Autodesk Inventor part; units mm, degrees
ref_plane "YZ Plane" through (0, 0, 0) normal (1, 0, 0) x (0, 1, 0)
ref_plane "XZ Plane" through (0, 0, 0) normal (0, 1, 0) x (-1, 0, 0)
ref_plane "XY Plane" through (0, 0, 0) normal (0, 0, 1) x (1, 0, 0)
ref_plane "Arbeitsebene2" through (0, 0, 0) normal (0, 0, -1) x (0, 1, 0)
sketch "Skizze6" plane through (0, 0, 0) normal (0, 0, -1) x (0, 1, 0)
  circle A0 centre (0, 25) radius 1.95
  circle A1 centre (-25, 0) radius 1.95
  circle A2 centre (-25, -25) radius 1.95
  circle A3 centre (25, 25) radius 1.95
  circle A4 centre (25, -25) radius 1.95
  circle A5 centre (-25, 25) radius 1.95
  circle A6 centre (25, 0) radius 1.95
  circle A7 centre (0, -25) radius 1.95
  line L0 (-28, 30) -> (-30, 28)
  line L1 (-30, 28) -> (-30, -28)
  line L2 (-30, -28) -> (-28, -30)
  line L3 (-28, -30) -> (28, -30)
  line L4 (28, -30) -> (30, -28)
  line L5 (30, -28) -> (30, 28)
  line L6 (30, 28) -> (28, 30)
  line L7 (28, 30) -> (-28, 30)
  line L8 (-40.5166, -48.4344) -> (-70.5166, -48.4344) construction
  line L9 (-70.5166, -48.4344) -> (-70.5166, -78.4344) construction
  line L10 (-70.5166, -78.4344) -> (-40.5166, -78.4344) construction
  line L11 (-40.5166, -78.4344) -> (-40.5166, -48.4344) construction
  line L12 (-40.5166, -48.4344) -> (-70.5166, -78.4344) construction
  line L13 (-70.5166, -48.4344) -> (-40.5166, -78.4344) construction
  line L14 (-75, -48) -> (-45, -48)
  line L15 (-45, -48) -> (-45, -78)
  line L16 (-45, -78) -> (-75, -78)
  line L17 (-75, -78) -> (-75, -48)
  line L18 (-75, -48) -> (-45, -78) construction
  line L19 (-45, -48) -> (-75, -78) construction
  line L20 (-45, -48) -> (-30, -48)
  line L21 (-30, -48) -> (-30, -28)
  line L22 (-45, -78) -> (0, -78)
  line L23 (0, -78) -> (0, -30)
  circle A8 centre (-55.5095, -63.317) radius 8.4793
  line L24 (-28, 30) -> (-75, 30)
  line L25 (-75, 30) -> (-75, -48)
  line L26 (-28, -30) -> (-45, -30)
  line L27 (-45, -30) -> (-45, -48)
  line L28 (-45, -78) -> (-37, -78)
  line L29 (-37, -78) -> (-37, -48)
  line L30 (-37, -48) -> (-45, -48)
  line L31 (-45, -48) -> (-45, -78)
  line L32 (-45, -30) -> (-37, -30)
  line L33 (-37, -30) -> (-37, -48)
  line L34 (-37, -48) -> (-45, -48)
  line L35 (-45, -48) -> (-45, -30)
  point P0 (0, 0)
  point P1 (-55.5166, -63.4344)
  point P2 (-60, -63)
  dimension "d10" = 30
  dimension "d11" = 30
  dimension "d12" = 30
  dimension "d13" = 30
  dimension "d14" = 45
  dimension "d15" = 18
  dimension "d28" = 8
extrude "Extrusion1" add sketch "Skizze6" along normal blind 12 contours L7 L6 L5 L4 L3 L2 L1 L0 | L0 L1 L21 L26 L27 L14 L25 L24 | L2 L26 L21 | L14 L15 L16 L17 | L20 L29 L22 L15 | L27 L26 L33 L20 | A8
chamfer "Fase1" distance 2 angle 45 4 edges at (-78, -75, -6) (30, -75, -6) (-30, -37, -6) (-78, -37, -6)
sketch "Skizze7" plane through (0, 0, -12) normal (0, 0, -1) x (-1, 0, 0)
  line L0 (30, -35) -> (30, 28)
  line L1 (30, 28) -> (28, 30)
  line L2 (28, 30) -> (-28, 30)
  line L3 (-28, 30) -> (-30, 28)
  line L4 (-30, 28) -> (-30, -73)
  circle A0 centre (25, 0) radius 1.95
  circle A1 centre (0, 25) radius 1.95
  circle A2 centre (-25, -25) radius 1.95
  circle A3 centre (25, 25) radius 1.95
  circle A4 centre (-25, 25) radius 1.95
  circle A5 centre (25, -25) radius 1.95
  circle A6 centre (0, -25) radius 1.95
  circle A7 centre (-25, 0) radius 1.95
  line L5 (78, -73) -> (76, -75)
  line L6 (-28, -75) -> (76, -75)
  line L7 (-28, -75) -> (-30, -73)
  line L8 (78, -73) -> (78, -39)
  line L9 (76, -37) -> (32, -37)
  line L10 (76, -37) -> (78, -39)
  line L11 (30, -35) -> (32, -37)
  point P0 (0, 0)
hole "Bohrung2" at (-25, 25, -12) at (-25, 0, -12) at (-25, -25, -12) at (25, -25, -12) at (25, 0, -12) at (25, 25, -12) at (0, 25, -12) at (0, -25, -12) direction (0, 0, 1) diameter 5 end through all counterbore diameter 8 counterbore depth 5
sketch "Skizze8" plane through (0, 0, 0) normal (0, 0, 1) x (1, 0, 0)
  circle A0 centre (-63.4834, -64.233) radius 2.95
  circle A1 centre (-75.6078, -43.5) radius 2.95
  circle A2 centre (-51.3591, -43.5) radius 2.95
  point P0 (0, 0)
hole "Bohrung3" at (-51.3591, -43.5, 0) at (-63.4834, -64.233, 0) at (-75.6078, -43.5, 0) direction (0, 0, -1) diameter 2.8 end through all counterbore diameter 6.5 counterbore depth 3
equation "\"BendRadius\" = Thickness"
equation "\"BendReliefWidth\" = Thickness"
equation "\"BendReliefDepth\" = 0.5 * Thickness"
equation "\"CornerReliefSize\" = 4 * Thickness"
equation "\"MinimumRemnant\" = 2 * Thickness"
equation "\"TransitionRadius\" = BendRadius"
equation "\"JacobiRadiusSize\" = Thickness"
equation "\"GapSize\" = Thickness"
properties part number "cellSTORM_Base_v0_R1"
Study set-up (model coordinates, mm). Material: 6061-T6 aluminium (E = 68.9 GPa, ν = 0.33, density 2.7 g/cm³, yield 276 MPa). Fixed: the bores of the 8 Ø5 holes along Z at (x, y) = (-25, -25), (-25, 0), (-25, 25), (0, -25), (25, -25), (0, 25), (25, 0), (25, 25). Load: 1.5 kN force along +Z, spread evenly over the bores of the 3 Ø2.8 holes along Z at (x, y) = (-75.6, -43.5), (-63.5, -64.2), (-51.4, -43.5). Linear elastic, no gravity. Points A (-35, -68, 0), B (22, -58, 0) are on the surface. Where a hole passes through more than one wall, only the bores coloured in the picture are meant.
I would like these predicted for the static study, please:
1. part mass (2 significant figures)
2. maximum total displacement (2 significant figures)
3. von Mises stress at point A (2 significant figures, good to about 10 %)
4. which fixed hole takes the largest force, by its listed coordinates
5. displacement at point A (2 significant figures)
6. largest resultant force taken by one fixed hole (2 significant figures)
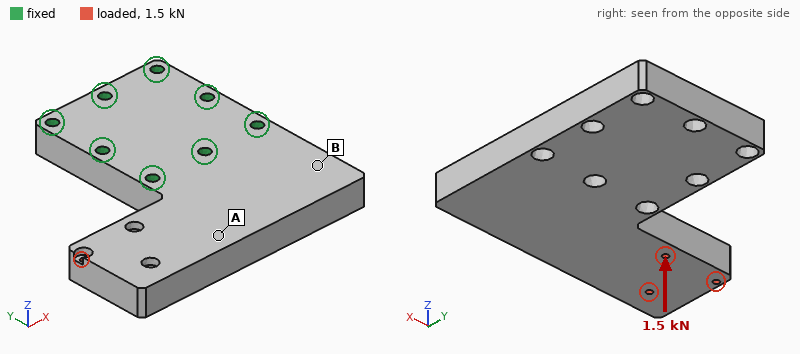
250 g
0.40 mm
38 MPa
(-25, -25)
0.14 mm
3.3 kN
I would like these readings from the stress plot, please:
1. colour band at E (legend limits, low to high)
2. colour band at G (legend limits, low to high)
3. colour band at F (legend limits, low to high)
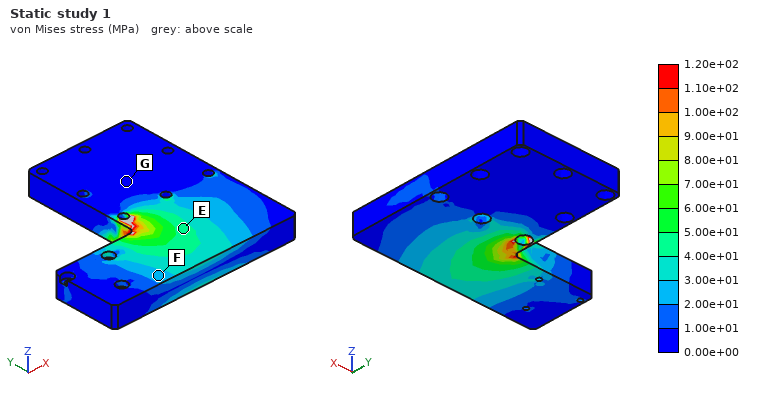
4.00e+01 to 5.00e+01 MPa
0.00e+00 to 1.00e+01 MPa
2.00e+01 to 3.00e+01 MPa
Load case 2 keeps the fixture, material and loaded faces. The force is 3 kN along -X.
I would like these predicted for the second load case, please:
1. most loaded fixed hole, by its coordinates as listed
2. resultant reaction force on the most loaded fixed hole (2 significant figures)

(-25, -25)
1.7 kN
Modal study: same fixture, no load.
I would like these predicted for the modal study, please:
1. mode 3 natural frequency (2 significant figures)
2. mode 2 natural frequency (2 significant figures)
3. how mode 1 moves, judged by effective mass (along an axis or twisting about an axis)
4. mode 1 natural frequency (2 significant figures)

4900 Hz
3100 Hz
along Z
1700 Hz
